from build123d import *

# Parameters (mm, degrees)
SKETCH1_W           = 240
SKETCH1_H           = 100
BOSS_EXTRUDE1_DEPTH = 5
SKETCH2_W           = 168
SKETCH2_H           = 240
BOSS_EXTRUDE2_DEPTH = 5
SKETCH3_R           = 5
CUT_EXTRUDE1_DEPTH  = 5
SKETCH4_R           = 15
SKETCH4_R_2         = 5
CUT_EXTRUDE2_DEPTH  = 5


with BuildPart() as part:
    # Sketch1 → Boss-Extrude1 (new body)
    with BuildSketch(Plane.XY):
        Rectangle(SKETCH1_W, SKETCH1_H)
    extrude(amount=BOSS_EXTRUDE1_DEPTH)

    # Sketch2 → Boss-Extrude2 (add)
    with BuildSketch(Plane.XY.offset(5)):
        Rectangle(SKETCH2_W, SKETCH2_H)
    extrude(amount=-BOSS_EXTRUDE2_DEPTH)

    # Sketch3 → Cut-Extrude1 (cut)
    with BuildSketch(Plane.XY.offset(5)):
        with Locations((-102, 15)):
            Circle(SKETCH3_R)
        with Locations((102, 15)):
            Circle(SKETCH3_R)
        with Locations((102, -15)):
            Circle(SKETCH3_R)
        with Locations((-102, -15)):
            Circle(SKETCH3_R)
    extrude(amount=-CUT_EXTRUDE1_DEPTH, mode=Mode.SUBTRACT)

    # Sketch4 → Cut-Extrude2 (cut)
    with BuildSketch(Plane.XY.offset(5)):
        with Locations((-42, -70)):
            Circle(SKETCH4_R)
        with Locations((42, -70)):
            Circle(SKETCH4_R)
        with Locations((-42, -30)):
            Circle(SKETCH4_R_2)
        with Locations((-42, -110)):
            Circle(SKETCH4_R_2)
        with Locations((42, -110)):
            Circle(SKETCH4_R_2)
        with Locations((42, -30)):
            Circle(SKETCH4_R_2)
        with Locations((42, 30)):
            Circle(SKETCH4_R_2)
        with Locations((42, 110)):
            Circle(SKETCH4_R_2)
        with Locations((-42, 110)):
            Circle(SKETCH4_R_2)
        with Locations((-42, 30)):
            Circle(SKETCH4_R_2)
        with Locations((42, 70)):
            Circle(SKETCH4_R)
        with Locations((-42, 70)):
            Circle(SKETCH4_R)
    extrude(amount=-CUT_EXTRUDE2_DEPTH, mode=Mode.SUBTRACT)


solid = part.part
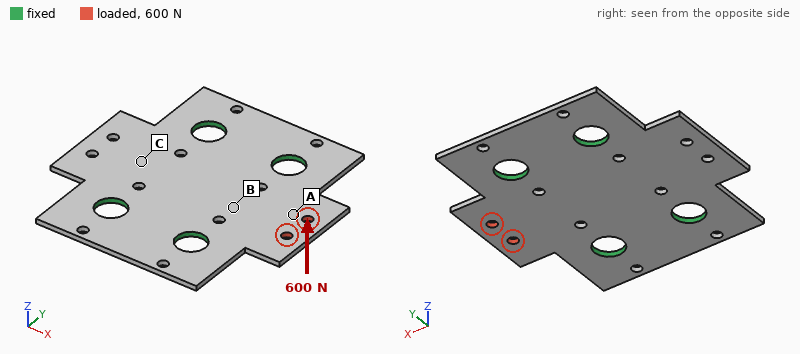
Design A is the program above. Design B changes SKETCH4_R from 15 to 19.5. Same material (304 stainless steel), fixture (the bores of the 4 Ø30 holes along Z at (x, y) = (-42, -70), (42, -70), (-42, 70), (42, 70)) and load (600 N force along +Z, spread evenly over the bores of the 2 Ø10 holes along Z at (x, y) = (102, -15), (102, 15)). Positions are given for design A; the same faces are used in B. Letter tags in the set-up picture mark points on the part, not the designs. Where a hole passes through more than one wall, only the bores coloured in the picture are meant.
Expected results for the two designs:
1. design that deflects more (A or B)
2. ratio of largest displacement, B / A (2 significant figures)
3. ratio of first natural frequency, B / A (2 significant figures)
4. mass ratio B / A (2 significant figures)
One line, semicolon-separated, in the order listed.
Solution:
A; 0.87; 1.1; 0.96
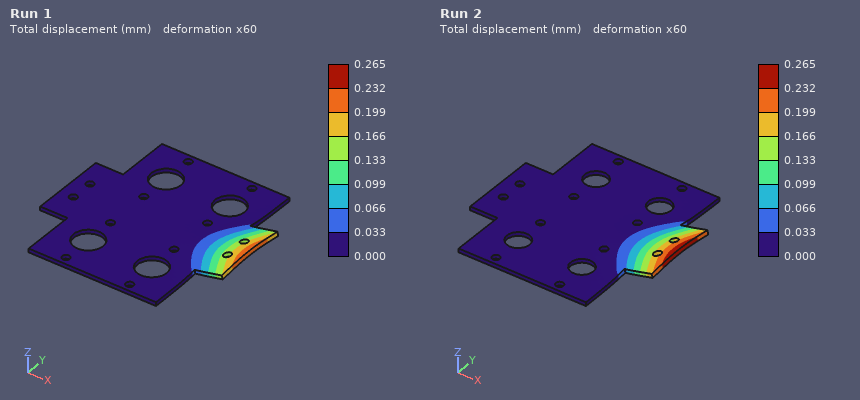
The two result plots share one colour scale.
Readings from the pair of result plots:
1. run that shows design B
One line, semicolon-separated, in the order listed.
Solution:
Run 1
